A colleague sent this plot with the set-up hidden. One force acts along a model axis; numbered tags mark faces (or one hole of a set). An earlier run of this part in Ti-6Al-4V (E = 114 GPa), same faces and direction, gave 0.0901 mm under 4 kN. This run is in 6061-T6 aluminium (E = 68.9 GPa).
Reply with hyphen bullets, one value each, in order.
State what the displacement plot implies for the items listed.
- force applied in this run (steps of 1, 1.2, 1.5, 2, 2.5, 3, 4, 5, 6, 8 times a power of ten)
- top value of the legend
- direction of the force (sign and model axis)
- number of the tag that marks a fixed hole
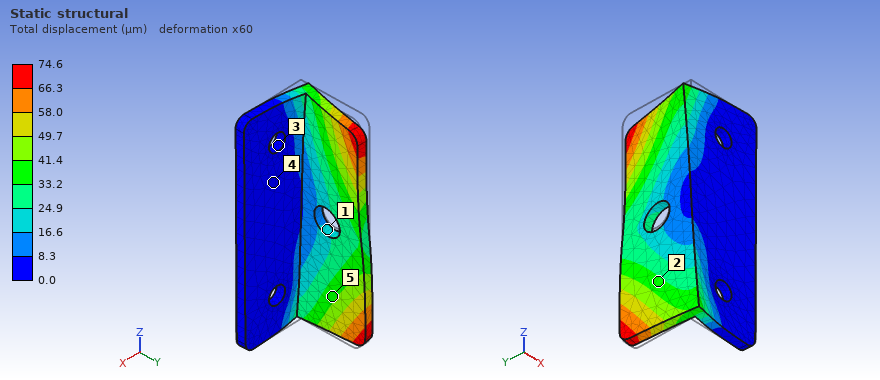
- 2 kN
- 74.6 µm
- -Z
- 3
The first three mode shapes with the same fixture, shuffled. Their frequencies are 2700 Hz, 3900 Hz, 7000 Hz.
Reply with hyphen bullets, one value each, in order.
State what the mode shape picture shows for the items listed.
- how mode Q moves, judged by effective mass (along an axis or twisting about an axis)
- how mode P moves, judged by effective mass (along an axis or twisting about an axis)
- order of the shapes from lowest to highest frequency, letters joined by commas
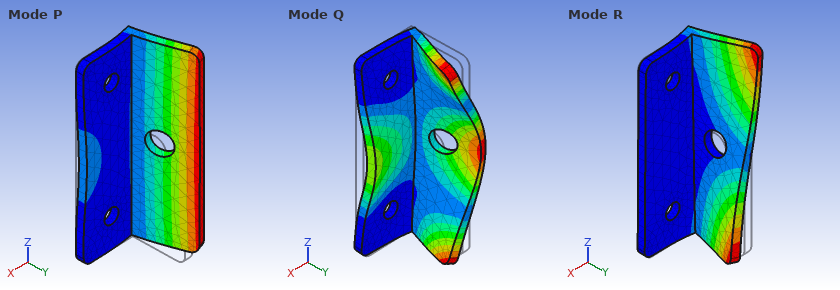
- along Y
- along X
- P, R, Q
